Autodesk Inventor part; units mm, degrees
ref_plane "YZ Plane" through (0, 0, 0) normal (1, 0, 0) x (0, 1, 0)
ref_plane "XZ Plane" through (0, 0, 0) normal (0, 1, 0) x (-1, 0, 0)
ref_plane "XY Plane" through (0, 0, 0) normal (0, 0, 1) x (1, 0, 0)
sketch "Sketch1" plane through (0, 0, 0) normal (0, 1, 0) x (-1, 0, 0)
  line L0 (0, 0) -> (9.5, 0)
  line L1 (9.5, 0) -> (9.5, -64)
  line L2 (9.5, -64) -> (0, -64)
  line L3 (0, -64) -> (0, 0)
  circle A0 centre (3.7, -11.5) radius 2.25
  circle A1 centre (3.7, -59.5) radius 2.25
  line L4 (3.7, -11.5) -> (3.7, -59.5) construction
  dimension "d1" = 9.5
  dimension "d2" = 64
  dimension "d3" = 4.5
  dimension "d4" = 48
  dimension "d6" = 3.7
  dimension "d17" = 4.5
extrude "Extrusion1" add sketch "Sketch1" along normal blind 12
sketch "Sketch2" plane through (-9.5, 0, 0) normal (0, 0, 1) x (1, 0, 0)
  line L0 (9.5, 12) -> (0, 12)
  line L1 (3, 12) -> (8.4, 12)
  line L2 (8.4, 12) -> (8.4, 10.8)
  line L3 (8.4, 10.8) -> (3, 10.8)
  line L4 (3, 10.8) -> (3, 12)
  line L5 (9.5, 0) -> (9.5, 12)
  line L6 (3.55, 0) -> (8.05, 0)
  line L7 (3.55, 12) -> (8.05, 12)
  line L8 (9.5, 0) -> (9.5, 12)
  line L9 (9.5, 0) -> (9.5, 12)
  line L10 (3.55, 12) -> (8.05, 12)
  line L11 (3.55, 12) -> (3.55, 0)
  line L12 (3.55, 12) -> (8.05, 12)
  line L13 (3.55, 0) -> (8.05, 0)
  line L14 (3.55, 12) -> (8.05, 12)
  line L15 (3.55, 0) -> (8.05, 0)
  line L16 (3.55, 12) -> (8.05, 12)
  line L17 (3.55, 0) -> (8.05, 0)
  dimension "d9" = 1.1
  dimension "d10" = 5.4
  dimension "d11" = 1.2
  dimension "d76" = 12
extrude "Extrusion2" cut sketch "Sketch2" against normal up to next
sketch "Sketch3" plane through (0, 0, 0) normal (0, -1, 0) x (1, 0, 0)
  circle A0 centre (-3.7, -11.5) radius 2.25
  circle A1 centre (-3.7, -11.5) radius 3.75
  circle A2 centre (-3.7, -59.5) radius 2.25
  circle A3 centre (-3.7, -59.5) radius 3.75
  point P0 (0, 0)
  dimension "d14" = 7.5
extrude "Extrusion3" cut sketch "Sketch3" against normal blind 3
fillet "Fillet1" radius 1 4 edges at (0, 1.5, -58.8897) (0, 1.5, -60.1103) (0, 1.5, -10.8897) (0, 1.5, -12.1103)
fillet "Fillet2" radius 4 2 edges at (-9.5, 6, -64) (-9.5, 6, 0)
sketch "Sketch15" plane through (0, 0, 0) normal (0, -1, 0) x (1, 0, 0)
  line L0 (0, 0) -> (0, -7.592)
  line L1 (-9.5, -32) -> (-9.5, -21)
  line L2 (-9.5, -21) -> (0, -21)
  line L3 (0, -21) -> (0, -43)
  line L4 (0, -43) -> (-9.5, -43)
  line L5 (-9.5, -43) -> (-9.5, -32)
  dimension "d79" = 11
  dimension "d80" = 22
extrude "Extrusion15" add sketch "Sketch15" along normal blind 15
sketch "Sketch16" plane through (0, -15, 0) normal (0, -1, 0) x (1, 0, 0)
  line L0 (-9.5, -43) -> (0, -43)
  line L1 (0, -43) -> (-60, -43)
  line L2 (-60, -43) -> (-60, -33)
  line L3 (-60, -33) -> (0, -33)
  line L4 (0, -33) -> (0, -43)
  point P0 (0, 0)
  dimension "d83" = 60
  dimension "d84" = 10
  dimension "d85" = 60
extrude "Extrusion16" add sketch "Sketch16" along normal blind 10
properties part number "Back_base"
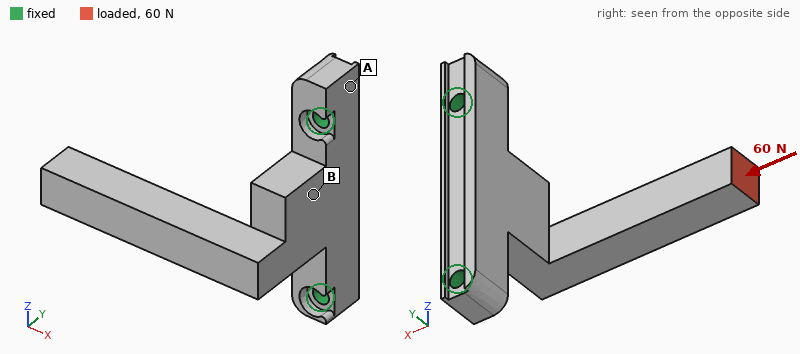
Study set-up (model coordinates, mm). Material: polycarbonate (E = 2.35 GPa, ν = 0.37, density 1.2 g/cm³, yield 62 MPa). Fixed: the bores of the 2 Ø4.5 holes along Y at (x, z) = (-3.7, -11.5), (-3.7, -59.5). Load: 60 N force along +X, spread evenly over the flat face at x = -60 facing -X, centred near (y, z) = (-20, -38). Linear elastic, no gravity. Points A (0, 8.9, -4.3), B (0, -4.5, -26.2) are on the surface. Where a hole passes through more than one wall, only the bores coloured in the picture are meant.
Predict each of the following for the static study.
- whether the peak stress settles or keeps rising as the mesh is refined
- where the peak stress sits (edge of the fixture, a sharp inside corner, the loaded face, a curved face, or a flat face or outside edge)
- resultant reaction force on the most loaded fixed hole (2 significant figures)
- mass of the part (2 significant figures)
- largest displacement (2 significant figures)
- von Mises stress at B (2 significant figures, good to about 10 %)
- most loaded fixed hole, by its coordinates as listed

keeps rising
edge of the fixture
34 N
18 g
1.0 mm
2.9 MPa
(-3.7, -59.5)
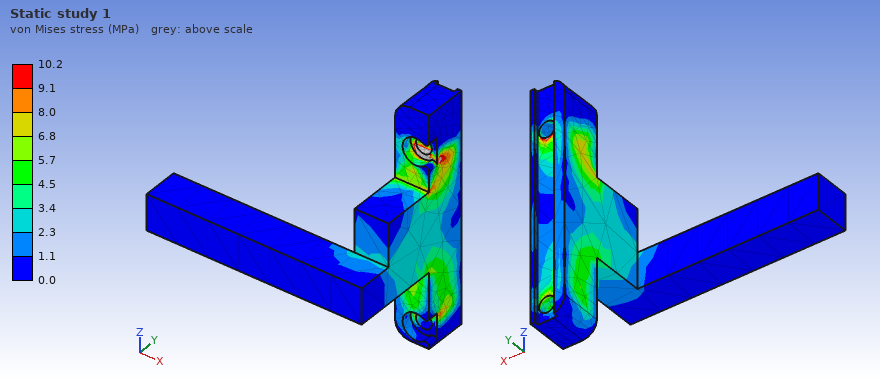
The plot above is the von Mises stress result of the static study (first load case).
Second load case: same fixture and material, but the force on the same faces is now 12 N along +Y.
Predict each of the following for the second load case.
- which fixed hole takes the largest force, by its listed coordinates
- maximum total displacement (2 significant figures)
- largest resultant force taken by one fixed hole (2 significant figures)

(-3.7, -59.5)
0.92 mm
7.9 N
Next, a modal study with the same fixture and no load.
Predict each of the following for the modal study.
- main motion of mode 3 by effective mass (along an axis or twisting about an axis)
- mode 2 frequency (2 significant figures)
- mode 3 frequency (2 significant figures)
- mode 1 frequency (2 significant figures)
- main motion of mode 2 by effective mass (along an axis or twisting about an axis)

along X
500 Hz
1100 Hz
380 Hz
along Z
